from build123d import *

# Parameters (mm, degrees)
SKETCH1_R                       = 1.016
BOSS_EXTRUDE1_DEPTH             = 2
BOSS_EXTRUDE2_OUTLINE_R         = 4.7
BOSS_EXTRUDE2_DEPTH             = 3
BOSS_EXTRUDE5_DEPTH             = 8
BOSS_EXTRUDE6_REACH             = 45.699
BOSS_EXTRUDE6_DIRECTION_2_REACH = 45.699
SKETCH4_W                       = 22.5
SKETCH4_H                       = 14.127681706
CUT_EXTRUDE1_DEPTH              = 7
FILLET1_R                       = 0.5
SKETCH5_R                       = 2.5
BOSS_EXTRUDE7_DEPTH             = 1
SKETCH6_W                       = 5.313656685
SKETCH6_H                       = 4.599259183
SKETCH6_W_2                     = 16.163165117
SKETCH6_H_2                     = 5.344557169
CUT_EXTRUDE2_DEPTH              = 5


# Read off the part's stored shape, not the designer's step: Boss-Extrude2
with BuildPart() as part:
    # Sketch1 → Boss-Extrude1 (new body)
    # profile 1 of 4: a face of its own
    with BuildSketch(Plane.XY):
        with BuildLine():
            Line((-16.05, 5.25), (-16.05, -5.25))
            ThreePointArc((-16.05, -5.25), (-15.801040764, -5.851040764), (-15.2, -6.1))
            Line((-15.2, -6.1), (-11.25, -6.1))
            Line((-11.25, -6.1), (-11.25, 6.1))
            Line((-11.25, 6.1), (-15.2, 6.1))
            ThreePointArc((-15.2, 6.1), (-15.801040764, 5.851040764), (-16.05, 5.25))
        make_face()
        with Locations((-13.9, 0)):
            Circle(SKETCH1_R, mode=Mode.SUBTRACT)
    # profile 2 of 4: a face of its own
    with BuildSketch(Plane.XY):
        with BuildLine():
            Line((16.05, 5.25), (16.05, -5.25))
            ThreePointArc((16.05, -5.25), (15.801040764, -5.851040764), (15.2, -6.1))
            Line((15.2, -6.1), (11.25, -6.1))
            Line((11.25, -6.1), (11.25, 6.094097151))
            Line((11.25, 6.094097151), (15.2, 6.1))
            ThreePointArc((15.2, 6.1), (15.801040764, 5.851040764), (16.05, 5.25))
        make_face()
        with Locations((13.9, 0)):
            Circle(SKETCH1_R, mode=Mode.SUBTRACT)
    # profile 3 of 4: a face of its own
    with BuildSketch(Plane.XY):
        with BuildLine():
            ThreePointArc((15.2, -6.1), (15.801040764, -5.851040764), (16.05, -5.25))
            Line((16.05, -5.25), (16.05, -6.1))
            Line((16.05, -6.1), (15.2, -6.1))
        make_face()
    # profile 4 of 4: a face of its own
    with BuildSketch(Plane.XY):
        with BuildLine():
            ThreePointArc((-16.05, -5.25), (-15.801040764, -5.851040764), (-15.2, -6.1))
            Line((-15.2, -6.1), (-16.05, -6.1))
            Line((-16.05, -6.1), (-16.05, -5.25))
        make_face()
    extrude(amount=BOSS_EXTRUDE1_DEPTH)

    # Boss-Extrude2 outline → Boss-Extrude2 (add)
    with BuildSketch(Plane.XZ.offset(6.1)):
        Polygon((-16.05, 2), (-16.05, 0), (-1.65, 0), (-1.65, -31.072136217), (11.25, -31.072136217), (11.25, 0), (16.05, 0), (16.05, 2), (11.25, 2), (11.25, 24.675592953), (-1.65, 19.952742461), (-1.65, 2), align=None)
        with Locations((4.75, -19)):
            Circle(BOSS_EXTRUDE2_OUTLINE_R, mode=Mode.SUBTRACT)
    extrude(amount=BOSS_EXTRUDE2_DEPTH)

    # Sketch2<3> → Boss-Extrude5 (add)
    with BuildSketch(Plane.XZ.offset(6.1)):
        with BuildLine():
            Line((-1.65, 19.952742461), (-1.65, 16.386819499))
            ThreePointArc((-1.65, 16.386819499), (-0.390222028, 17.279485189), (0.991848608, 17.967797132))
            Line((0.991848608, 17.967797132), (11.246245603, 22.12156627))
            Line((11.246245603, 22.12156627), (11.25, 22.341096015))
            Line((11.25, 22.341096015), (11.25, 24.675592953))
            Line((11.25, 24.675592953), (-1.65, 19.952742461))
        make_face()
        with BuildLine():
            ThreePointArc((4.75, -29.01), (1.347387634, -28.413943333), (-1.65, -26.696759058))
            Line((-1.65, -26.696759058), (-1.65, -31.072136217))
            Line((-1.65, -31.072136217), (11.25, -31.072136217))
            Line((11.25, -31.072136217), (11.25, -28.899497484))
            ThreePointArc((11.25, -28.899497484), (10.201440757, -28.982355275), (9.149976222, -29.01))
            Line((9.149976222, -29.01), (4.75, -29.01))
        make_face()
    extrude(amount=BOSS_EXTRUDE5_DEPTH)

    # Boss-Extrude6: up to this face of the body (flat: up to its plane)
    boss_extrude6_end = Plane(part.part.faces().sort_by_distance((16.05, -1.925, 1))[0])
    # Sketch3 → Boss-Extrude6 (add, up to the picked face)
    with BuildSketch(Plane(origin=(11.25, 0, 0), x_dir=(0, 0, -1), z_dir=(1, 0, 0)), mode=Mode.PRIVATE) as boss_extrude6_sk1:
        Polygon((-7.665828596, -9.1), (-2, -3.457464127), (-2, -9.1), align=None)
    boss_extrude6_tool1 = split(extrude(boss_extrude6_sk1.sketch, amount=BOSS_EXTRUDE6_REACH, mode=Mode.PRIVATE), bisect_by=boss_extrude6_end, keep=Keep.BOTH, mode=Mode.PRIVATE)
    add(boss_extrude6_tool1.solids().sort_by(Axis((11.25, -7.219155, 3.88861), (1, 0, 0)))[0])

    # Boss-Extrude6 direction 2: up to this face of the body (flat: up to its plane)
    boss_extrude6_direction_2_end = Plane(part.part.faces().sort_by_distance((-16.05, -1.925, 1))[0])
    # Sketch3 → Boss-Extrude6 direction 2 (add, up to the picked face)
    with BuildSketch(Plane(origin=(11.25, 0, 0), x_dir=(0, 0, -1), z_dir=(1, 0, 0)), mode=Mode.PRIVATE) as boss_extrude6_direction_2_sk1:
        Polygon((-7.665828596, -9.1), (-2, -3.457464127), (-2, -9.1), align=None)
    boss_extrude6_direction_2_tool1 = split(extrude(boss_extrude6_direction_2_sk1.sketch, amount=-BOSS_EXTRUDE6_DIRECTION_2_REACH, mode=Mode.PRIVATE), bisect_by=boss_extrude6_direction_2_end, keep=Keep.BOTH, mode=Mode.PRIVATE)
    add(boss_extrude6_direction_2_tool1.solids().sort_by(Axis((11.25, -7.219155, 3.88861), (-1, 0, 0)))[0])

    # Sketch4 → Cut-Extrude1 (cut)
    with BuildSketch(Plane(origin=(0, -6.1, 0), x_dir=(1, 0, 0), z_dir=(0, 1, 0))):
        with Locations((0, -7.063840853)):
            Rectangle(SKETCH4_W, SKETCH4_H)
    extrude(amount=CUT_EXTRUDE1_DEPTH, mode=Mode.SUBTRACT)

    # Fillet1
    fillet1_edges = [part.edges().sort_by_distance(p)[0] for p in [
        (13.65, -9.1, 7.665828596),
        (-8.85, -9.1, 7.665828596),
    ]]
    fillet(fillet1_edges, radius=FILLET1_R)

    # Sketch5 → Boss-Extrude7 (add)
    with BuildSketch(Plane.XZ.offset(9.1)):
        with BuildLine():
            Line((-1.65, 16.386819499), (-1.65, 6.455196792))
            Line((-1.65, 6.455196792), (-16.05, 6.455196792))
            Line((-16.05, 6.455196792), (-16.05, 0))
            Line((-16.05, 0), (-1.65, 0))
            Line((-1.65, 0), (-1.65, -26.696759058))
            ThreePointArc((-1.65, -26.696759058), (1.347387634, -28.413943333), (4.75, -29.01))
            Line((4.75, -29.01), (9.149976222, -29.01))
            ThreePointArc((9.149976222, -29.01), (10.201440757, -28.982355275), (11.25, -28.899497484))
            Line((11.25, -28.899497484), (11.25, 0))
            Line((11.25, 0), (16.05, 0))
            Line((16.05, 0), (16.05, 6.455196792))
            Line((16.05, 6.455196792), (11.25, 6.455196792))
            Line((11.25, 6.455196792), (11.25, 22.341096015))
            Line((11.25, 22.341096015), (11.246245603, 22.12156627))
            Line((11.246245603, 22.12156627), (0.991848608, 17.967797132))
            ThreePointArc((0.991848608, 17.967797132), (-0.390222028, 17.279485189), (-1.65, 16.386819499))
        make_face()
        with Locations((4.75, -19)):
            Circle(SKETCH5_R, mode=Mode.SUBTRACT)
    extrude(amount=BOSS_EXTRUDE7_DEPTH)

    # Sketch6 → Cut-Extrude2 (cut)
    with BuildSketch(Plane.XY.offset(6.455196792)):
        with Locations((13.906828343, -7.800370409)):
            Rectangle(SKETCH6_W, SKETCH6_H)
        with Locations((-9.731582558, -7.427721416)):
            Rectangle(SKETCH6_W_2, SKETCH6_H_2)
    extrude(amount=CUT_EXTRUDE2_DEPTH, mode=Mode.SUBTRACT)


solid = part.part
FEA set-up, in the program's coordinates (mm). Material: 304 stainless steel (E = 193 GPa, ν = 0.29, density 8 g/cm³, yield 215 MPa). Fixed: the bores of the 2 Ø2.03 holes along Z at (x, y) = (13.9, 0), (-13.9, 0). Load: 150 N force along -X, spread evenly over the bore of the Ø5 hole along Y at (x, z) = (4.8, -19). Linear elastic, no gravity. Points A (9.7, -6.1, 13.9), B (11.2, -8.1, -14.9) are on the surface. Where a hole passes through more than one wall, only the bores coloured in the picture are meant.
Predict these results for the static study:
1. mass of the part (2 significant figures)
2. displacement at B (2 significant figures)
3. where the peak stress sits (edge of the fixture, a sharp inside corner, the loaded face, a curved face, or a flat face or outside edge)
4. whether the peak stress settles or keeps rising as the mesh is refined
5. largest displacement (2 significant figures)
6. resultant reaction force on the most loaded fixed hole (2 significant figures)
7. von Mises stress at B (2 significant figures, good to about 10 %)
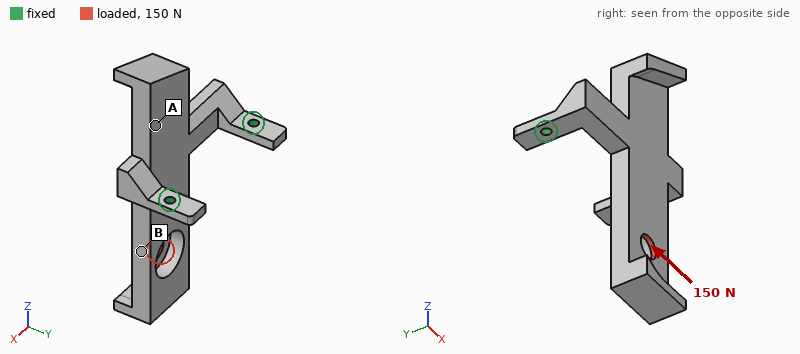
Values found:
28 g
21 µm
edge of the fixture
keeps rising
41 µm
140 N
14 MPa
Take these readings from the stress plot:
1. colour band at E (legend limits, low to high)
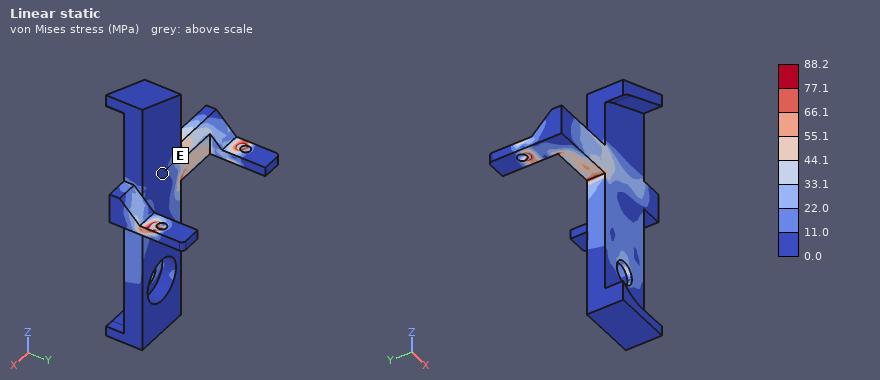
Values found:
0.0 to 11.0 MPa
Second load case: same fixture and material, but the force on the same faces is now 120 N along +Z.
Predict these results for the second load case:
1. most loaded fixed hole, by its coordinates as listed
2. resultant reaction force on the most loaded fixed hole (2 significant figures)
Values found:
(13.9, 0)
79 N
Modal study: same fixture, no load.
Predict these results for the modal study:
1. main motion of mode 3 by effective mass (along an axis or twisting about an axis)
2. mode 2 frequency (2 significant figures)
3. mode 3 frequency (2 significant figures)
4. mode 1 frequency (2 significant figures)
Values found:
along Y
3300 Hz
3700 Hz
890 Hz
